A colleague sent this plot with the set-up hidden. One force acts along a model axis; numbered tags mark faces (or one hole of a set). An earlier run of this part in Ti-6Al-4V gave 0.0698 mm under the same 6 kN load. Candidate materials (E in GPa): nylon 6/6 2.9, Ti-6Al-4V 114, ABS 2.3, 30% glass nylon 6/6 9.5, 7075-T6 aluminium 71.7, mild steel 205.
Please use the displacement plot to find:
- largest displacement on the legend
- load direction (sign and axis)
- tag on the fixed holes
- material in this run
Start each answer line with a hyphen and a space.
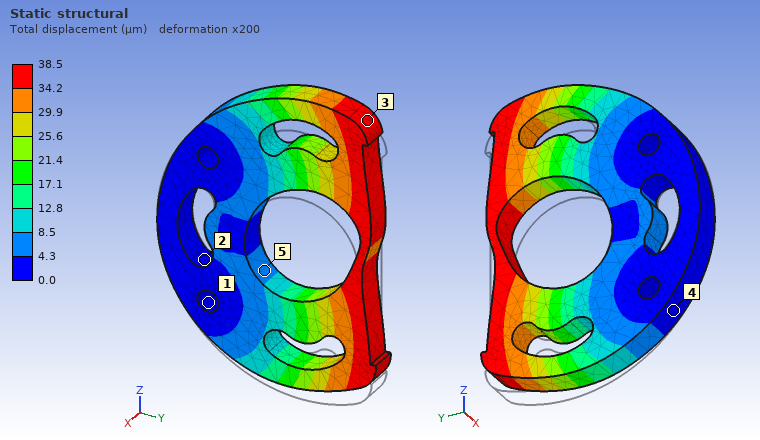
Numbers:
- 38.5 µm
- +Z
- 1
- mild steel
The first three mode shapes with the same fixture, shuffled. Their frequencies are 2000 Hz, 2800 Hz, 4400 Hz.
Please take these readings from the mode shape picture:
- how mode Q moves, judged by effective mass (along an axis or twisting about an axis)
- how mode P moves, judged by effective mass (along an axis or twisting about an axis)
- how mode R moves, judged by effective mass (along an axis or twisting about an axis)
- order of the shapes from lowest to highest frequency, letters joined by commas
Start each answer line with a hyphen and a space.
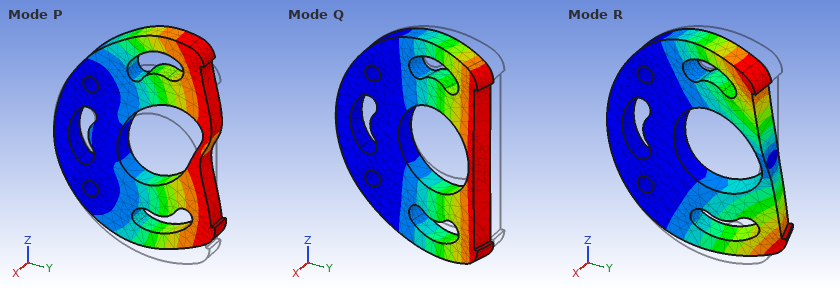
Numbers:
- along X
- along Z
- twisting about Y
- Q, R, P
